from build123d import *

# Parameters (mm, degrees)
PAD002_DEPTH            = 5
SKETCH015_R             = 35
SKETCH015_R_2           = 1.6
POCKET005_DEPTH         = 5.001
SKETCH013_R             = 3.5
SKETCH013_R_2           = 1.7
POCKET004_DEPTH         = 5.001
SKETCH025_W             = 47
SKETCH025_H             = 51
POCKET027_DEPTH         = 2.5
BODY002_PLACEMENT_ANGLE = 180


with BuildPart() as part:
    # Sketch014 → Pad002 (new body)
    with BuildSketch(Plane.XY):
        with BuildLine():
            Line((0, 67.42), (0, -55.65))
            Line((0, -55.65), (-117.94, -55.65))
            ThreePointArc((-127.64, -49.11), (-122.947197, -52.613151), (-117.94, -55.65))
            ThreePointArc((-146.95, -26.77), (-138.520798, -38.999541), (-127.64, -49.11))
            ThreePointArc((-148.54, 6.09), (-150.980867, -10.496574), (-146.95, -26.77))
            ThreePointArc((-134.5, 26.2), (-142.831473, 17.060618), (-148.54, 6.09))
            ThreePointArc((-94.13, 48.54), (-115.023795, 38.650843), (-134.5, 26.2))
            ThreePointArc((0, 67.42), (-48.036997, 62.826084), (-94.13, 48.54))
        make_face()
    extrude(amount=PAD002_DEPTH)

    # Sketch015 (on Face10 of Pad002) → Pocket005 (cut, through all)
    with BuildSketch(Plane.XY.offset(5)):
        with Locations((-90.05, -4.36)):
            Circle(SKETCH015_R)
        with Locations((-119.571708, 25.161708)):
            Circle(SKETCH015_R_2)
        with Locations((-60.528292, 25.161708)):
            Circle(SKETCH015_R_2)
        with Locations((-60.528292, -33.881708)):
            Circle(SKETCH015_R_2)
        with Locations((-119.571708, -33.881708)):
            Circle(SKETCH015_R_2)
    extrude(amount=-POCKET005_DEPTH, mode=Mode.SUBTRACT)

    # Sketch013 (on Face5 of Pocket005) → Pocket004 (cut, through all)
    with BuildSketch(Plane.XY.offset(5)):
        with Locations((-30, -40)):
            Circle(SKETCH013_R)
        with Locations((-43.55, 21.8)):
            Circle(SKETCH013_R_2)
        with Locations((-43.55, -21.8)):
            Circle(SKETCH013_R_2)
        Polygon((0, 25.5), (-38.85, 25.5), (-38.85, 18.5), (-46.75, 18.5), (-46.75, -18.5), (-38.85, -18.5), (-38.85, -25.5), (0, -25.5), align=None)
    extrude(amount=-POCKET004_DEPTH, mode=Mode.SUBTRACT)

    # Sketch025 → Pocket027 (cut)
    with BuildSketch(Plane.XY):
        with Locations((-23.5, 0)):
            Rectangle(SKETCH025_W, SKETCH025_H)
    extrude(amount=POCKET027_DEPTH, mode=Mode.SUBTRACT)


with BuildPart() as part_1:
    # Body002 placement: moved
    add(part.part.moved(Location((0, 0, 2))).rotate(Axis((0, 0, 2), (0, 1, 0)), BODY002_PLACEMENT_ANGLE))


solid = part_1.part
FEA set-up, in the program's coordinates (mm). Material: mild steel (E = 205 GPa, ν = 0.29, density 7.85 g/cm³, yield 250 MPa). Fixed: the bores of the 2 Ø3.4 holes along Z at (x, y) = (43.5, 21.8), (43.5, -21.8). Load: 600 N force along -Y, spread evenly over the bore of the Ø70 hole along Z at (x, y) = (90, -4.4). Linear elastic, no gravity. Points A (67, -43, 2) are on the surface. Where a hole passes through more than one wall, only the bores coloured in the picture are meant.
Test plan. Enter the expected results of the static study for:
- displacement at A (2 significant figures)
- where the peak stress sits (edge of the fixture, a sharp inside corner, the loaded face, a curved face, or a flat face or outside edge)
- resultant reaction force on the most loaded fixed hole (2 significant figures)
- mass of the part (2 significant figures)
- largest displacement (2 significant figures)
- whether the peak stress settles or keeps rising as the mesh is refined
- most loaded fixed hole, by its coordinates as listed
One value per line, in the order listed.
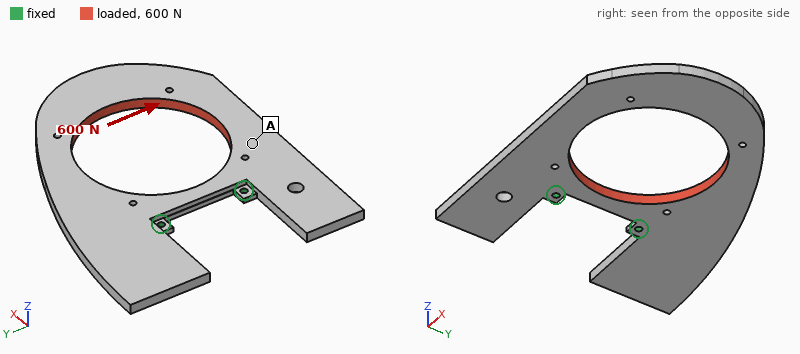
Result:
19 µm
edge of the fixture
600 N
360 g
51 µm
keeps rising
(43.5, -21.8)
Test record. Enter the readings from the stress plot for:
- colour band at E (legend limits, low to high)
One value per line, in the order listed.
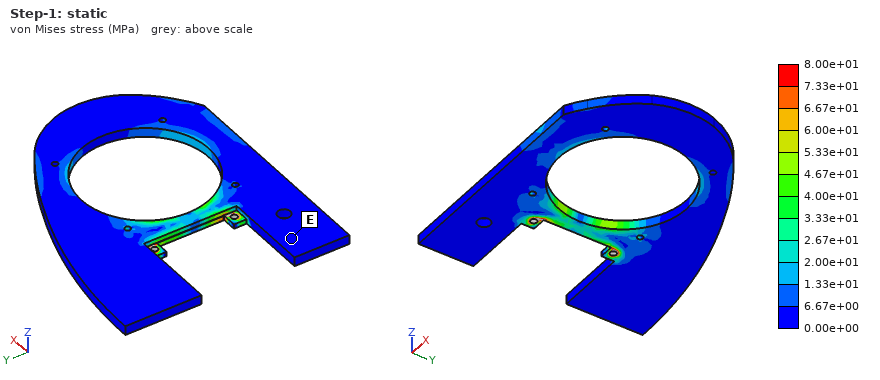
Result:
0.00e+00 to 6.67e+00 MPa
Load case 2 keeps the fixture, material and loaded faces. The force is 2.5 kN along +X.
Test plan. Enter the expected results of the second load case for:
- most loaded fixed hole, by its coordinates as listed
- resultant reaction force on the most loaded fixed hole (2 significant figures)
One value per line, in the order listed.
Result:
(43.5, -21.8)
1.5 kN
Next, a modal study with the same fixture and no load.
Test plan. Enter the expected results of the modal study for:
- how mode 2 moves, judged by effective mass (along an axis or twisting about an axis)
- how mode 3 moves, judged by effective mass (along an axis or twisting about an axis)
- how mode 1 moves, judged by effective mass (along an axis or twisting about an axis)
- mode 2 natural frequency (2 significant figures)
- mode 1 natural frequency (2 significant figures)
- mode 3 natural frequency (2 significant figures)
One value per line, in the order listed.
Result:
twisting about X
along Z
along Z
650 Hz
230 Hz
850 Hz
